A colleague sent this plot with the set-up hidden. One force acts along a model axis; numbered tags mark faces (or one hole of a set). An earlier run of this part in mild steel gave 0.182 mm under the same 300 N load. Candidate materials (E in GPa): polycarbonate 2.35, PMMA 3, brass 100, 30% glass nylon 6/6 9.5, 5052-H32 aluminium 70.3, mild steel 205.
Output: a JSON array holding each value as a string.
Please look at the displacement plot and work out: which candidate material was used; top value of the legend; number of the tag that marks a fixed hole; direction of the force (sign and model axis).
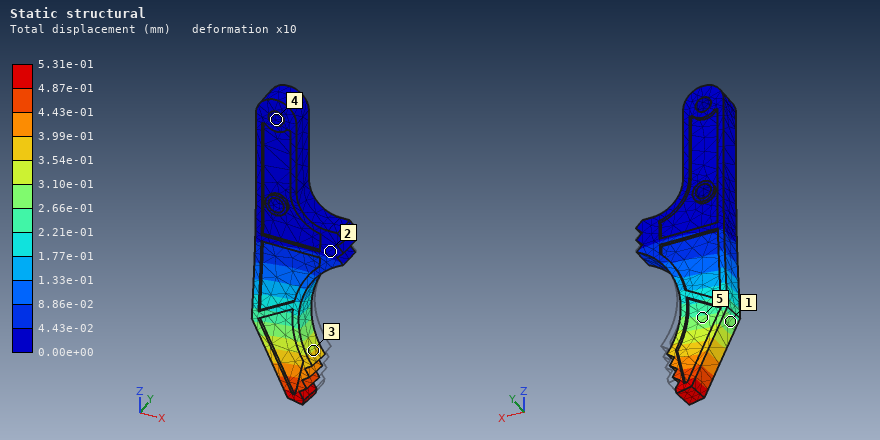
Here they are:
["5052-H32 aluminium", "5.31e-01 mm", "4", "-Y"]
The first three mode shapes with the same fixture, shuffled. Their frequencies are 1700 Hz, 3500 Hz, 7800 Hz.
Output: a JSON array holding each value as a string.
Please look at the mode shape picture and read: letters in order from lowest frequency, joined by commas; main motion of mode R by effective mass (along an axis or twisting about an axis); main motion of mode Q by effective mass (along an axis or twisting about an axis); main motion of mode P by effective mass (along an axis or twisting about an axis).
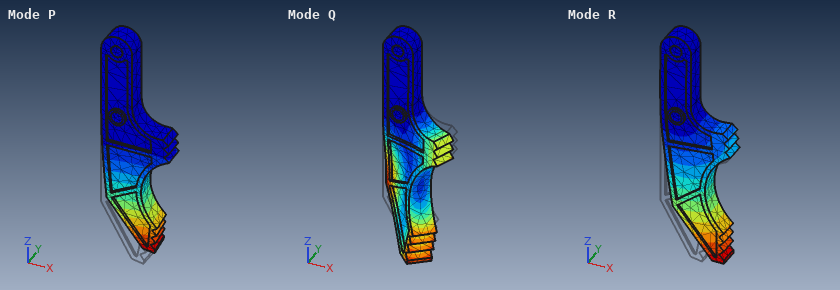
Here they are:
["P, R, Q", "along X", "twisting about Z", "along Y"]
